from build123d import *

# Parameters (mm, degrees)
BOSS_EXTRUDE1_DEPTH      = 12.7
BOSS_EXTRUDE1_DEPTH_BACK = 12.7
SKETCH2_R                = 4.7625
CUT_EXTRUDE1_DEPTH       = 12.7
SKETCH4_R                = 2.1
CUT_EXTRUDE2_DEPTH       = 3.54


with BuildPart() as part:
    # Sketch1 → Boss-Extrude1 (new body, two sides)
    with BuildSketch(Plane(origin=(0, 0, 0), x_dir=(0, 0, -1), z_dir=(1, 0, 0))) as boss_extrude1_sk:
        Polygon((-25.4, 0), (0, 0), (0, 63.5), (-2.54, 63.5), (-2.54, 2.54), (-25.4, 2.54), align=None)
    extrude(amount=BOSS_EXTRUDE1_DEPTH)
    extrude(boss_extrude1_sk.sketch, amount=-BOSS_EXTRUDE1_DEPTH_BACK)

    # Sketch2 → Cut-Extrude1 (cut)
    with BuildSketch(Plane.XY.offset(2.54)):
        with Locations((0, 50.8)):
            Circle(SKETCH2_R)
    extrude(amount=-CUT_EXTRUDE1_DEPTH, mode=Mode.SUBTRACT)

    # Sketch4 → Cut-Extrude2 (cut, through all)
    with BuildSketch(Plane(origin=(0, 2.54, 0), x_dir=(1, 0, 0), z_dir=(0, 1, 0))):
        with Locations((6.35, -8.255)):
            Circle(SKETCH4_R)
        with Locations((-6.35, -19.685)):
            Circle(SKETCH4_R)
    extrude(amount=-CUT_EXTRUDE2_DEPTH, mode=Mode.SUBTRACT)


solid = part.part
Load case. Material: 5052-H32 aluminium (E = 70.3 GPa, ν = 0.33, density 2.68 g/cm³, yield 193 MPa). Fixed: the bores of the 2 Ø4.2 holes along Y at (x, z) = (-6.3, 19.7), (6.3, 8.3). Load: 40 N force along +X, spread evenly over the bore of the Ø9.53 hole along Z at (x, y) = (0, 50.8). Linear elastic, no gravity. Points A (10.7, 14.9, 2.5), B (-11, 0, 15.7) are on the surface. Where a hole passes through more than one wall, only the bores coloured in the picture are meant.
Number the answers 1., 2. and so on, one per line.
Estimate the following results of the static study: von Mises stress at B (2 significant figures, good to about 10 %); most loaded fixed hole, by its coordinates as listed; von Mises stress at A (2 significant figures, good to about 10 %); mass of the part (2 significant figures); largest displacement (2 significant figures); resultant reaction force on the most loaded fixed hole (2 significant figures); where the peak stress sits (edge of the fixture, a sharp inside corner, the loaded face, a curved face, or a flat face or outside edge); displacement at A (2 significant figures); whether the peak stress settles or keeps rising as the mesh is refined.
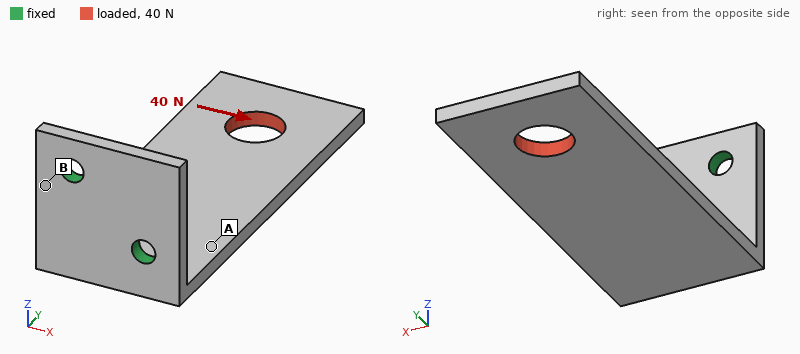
1. 30 MPa
2. (6.3, 8.3)
3. 8.7 MPa
4. 14 g
5. 0.20 mm
6. 58 N
7. edge of the fixture
8. 0.040 mm
9. keeps rising
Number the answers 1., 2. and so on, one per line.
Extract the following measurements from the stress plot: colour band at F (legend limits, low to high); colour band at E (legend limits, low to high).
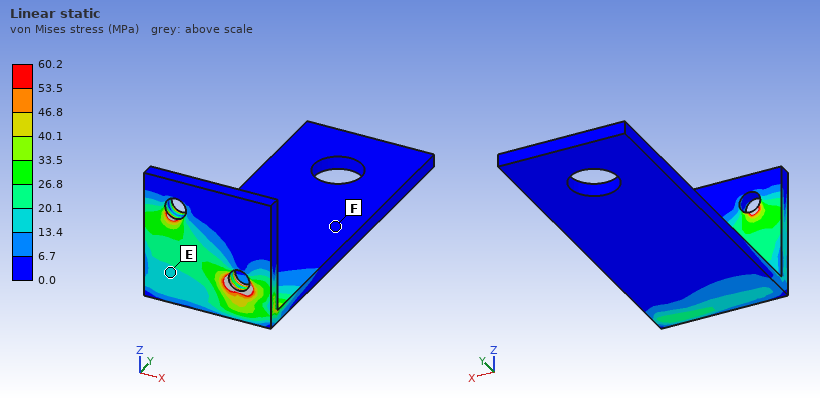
1. 0.0 to 6.7 MPa
2. 13.4 to 20.1 MPa
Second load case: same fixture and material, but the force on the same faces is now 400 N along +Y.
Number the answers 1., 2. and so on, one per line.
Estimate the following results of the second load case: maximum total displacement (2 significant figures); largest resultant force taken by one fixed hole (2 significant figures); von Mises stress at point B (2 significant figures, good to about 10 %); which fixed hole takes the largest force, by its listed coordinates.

1. 0.40 mm
2. 370 N
3. 46 MPa
4. (6.3, 8.3)
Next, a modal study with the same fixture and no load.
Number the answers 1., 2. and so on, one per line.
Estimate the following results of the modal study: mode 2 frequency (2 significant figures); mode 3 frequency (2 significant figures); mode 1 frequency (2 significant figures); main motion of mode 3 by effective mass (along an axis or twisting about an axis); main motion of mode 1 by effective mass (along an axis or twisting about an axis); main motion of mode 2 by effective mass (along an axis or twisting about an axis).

1. 1200 Hz
2. 2600 Hz
3. 490 Hz
4. twisting about Y
5. along Z
6. along X
